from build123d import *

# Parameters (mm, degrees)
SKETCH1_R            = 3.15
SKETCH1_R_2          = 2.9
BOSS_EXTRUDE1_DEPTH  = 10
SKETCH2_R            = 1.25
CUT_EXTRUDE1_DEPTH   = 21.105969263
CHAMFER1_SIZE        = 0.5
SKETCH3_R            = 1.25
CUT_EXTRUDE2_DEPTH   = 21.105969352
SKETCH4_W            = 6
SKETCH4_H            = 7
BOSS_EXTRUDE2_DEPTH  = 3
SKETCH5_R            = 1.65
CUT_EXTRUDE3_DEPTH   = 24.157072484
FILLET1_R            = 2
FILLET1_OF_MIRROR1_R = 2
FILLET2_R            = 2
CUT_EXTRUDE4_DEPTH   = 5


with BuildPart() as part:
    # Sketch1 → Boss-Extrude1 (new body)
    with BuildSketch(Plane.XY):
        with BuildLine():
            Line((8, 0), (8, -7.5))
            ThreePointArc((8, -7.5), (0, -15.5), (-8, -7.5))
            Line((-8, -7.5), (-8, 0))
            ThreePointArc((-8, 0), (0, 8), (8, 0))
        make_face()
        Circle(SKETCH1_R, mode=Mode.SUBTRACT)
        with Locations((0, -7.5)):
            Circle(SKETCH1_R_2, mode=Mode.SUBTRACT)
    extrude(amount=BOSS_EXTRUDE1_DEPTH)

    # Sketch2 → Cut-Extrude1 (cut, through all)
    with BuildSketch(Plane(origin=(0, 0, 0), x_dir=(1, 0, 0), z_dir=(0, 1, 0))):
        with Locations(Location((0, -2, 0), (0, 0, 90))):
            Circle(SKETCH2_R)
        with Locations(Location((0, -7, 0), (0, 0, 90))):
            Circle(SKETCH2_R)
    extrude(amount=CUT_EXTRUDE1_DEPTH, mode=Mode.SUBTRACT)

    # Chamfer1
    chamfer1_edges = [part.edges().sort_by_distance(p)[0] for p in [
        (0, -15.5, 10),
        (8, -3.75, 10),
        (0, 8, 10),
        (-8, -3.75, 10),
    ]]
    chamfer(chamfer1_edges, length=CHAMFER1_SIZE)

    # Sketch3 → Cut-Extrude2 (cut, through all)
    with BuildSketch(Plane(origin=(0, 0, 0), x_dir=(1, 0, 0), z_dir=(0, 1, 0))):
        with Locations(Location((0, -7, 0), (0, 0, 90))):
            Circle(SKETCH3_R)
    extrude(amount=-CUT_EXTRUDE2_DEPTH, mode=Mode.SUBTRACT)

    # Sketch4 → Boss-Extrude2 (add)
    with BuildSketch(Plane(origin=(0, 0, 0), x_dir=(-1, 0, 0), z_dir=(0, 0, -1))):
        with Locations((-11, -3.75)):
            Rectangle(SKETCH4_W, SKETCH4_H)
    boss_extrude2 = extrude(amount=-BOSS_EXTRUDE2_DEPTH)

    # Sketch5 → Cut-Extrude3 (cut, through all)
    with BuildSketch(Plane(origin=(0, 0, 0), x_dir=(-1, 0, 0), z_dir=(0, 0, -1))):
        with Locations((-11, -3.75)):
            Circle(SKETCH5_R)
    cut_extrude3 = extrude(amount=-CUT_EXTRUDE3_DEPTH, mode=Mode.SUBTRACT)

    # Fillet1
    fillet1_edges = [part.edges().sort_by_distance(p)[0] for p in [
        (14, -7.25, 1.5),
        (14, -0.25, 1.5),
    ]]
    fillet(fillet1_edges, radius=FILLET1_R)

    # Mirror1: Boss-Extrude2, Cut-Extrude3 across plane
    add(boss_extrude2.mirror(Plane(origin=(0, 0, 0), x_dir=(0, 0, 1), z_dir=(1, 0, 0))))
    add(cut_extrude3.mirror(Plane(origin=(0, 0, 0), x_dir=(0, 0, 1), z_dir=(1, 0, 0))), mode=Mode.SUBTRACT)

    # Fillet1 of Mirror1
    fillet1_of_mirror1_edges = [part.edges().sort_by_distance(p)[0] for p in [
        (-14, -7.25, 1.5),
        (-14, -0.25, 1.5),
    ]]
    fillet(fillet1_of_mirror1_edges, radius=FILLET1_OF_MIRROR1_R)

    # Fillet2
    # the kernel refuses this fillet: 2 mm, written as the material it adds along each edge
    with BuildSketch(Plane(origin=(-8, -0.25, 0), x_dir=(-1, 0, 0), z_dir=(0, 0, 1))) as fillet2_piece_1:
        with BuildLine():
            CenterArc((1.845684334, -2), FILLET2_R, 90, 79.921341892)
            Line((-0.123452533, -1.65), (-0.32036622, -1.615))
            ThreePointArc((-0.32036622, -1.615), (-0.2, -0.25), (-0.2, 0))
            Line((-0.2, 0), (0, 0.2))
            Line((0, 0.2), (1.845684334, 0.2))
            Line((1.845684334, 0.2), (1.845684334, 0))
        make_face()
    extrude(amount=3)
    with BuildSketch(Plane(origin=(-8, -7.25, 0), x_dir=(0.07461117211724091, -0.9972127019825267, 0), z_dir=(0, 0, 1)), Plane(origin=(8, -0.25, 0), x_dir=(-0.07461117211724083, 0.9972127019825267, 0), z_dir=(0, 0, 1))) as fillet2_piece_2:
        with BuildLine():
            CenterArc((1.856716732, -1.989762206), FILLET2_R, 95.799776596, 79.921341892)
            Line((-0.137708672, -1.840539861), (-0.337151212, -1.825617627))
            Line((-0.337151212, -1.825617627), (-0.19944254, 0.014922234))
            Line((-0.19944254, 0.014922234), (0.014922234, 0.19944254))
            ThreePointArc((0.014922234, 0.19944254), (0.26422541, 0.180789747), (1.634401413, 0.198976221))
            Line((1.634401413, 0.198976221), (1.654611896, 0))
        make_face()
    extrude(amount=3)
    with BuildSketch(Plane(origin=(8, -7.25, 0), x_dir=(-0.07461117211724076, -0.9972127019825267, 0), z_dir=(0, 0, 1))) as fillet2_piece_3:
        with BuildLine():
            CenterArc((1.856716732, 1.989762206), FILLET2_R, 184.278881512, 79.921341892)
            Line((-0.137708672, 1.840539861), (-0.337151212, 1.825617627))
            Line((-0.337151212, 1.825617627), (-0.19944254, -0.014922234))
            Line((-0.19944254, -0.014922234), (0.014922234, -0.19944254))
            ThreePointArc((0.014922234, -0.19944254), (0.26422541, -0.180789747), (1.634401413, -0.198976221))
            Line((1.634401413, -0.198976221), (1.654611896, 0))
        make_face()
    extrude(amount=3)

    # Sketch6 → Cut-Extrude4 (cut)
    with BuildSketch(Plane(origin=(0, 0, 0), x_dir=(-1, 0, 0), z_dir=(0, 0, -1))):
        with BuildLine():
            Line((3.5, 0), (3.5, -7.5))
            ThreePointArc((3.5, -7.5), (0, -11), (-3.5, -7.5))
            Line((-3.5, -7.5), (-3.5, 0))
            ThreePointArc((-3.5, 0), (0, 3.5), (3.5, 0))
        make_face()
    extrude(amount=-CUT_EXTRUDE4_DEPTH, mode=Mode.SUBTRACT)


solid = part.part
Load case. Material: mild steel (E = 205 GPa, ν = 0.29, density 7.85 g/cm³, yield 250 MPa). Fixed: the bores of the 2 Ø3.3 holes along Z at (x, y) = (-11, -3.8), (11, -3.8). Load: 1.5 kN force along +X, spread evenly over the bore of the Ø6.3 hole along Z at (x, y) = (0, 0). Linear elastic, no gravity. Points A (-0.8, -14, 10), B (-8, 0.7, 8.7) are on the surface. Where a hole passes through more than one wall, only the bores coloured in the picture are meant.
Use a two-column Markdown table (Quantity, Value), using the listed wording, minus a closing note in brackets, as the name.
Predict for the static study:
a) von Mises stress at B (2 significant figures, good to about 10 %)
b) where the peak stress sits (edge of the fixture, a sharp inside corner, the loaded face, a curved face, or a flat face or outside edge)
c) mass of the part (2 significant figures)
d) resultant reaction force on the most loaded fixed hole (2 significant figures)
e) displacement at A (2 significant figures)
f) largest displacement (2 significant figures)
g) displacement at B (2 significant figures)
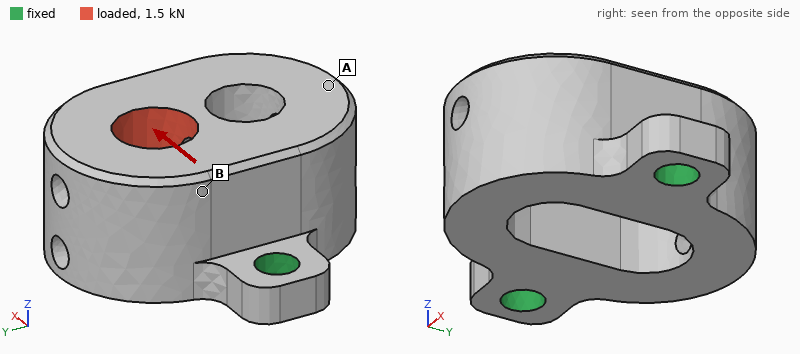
| Quantity | Value |
|---|---|
| von Mises stress at B | 18 MPa |
| where the peak stress sits | a curved face |
| mass of the part | 20 g |
| resultant reaction force on the most loaded fixed hole | 930 N |
| displacement at A | 1.5 µm |
| largest displacement | 4.8 µm |
| displacement at B | 4.2 µm |
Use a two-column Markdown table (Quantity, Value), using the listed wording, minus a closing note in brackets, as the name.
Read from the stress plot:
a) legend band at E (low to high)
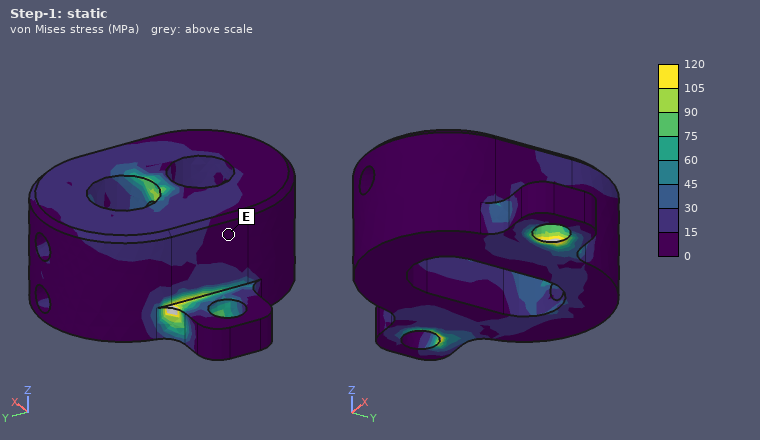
| Quantity | Value |
|---|---|
| legend band at E | 0 to 15 MPa |
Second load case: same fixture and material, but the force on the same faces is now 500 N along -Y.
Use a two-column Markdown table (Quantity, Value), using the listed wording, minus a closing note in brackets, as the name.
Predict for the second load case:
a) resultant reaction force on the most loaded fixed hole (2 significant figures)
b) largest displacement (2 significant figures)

| Quantity | Value |
|---|---|
| resultant reaction force on the most loaded fixed hole | 250 N |
| largest displacement | 13 µm |
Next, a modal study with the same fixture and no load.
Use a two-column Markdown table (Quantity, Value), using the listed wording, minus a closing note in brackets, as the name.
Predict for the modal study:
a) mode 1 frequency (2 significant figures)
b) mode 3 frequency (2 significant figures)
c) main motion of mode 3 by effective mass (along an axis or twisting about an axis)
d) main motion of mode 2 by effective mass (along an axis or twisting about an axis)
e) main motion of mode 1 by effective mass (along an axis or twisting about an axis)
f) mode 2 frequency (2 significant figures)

| Quantity | Value |
|---|---|
| mode 1 frequency | 8700 Hz |
| mode 3 frequency | 33 kHz |
| main motion of mode 3 by effective mass | along X |
| main motion of mode 2 by effective mass | along Z |
| main motion of mode 1 by effective mass | along Y |
| mode 2 frequency | 25 kHz |
